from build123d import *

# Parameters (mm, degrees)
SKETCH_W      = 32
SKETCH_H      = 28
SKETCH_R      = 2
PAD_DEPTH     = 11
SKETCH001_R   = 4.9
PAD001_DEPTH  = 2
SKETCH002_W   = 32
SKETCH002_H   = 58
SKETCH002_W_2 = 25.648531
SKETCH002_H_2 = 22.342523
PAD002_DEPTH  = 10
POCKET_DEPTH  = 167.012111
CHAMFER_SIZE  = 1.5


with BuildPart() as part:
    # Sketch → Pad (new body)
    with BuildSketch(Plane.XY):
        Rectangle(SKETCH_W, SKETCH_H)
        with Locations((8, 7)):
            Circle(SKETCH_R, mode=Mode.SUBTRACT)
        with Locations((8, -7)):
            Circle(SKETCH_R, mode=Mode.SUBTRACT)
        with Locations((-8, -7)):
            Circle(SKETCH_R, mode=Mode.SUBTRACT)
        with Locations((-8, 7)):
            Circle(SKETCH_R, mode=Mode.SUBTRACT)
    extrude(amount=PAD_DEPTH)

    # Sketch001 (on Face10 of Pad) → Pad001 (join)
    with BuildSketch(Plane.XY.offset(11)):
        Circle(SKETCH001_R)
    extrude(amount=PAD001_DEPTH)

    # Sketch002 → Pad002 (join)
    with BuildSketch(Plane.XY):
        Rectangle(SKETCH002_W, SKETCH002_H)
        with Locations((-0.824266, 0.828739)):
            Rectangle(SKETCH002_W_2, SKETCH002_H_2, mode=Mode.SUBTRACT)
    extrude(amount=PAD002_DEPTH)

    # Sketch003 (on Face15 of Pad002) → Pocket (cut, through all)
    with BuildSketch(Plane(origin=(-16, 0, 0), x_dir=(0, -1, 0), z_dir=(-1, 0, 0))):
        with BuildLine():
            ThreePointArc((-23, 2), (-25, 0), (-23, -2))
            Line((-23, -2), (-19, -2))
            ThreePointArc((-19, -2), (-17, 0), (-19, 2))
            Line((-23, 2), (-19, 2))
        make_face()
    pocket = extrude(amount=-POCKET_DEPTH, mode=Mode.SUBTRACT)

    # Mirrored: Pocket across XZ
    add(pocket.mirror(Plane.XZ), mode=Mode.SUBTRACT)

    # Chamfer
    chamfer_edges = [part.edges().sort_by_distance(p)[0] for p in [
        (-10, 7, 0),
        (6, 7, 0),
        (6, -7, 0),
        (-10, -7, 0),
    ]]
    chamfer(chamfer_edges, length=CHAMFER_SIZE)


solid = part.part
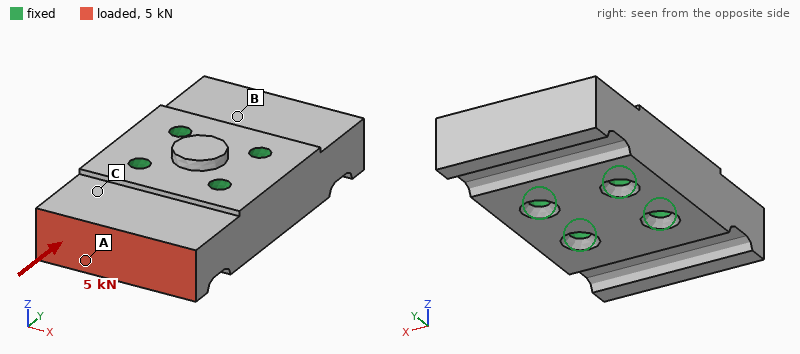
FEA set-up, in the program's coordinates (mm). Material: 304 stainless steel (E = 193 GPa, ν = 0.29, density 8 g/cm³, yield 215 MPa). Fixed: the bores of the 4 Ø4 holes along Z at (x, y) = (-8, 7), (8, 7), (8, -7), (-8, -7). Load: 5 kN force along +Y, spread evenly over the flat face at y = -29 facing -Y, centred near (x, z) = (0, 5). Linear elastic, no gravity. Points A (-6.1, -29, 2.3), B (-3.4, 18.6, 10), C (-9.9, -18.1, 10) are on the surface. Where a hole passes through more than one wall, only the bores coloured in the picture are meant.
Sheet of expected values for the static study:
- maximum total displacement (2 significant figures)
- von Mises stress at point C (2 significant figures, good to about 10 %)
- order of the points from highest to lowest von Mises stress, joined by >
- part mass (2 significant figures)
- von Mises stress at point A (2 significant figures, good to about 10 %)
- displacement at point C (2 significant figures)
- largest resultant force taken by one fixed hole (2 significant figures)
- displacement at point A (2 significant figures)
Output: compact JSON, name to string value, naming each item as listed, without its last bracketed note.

{"maximum total displacement": "4.2 µm", "von Mises stress at point C": "10.0 MPa", "order of the points from highest to lowest von Mises stress, joined by >": "A > C > B", "part mass": "140 g", "von Mises stress at point A": "19 MPa", "displacement at point C": "0.80 µm", "largest resultant force taken by one fixed hole": "2.1 kN", "displacement at point A": "3.7 µm"}
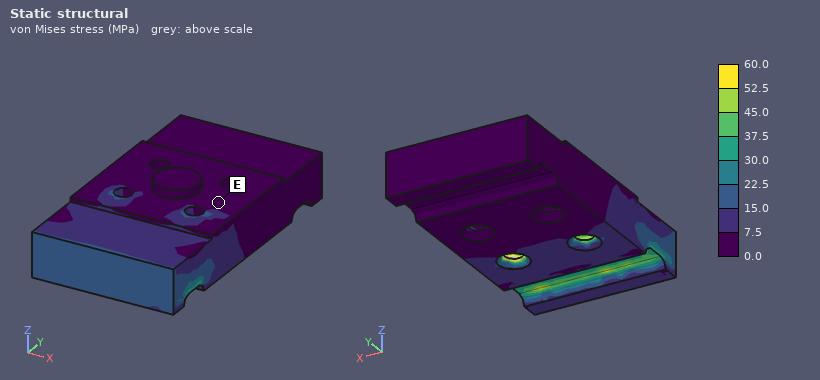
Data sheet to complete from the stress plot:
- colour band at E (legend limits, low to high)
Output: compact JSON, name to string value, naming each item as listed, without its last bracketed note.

{"colour band at E": "0.0 to 7.5 MPa"}
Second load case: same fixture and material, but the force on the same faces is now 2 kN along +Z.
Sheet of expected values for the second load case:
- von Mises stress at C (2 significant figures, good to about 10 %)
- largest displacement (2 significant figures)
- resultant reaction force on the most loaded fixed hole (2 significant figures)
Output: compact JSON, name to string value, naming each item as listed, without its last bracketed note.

{"von Mises stress at C": "54 MPa", "largest displacement": "19 µm", "resultant reaction force on the most loaded fixed hole": "1.4 kN"}
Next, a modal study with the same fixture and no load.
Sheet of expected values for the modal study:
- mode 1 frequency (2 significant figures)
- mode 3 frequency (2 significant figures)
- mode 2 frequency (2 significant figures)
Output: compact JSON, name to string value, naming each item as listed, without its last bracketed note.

{"mode 1 frequency": "15 kHz", "mode 3 frequency": "22 kHz", "mode 2 frequency": "15 kHz"}
